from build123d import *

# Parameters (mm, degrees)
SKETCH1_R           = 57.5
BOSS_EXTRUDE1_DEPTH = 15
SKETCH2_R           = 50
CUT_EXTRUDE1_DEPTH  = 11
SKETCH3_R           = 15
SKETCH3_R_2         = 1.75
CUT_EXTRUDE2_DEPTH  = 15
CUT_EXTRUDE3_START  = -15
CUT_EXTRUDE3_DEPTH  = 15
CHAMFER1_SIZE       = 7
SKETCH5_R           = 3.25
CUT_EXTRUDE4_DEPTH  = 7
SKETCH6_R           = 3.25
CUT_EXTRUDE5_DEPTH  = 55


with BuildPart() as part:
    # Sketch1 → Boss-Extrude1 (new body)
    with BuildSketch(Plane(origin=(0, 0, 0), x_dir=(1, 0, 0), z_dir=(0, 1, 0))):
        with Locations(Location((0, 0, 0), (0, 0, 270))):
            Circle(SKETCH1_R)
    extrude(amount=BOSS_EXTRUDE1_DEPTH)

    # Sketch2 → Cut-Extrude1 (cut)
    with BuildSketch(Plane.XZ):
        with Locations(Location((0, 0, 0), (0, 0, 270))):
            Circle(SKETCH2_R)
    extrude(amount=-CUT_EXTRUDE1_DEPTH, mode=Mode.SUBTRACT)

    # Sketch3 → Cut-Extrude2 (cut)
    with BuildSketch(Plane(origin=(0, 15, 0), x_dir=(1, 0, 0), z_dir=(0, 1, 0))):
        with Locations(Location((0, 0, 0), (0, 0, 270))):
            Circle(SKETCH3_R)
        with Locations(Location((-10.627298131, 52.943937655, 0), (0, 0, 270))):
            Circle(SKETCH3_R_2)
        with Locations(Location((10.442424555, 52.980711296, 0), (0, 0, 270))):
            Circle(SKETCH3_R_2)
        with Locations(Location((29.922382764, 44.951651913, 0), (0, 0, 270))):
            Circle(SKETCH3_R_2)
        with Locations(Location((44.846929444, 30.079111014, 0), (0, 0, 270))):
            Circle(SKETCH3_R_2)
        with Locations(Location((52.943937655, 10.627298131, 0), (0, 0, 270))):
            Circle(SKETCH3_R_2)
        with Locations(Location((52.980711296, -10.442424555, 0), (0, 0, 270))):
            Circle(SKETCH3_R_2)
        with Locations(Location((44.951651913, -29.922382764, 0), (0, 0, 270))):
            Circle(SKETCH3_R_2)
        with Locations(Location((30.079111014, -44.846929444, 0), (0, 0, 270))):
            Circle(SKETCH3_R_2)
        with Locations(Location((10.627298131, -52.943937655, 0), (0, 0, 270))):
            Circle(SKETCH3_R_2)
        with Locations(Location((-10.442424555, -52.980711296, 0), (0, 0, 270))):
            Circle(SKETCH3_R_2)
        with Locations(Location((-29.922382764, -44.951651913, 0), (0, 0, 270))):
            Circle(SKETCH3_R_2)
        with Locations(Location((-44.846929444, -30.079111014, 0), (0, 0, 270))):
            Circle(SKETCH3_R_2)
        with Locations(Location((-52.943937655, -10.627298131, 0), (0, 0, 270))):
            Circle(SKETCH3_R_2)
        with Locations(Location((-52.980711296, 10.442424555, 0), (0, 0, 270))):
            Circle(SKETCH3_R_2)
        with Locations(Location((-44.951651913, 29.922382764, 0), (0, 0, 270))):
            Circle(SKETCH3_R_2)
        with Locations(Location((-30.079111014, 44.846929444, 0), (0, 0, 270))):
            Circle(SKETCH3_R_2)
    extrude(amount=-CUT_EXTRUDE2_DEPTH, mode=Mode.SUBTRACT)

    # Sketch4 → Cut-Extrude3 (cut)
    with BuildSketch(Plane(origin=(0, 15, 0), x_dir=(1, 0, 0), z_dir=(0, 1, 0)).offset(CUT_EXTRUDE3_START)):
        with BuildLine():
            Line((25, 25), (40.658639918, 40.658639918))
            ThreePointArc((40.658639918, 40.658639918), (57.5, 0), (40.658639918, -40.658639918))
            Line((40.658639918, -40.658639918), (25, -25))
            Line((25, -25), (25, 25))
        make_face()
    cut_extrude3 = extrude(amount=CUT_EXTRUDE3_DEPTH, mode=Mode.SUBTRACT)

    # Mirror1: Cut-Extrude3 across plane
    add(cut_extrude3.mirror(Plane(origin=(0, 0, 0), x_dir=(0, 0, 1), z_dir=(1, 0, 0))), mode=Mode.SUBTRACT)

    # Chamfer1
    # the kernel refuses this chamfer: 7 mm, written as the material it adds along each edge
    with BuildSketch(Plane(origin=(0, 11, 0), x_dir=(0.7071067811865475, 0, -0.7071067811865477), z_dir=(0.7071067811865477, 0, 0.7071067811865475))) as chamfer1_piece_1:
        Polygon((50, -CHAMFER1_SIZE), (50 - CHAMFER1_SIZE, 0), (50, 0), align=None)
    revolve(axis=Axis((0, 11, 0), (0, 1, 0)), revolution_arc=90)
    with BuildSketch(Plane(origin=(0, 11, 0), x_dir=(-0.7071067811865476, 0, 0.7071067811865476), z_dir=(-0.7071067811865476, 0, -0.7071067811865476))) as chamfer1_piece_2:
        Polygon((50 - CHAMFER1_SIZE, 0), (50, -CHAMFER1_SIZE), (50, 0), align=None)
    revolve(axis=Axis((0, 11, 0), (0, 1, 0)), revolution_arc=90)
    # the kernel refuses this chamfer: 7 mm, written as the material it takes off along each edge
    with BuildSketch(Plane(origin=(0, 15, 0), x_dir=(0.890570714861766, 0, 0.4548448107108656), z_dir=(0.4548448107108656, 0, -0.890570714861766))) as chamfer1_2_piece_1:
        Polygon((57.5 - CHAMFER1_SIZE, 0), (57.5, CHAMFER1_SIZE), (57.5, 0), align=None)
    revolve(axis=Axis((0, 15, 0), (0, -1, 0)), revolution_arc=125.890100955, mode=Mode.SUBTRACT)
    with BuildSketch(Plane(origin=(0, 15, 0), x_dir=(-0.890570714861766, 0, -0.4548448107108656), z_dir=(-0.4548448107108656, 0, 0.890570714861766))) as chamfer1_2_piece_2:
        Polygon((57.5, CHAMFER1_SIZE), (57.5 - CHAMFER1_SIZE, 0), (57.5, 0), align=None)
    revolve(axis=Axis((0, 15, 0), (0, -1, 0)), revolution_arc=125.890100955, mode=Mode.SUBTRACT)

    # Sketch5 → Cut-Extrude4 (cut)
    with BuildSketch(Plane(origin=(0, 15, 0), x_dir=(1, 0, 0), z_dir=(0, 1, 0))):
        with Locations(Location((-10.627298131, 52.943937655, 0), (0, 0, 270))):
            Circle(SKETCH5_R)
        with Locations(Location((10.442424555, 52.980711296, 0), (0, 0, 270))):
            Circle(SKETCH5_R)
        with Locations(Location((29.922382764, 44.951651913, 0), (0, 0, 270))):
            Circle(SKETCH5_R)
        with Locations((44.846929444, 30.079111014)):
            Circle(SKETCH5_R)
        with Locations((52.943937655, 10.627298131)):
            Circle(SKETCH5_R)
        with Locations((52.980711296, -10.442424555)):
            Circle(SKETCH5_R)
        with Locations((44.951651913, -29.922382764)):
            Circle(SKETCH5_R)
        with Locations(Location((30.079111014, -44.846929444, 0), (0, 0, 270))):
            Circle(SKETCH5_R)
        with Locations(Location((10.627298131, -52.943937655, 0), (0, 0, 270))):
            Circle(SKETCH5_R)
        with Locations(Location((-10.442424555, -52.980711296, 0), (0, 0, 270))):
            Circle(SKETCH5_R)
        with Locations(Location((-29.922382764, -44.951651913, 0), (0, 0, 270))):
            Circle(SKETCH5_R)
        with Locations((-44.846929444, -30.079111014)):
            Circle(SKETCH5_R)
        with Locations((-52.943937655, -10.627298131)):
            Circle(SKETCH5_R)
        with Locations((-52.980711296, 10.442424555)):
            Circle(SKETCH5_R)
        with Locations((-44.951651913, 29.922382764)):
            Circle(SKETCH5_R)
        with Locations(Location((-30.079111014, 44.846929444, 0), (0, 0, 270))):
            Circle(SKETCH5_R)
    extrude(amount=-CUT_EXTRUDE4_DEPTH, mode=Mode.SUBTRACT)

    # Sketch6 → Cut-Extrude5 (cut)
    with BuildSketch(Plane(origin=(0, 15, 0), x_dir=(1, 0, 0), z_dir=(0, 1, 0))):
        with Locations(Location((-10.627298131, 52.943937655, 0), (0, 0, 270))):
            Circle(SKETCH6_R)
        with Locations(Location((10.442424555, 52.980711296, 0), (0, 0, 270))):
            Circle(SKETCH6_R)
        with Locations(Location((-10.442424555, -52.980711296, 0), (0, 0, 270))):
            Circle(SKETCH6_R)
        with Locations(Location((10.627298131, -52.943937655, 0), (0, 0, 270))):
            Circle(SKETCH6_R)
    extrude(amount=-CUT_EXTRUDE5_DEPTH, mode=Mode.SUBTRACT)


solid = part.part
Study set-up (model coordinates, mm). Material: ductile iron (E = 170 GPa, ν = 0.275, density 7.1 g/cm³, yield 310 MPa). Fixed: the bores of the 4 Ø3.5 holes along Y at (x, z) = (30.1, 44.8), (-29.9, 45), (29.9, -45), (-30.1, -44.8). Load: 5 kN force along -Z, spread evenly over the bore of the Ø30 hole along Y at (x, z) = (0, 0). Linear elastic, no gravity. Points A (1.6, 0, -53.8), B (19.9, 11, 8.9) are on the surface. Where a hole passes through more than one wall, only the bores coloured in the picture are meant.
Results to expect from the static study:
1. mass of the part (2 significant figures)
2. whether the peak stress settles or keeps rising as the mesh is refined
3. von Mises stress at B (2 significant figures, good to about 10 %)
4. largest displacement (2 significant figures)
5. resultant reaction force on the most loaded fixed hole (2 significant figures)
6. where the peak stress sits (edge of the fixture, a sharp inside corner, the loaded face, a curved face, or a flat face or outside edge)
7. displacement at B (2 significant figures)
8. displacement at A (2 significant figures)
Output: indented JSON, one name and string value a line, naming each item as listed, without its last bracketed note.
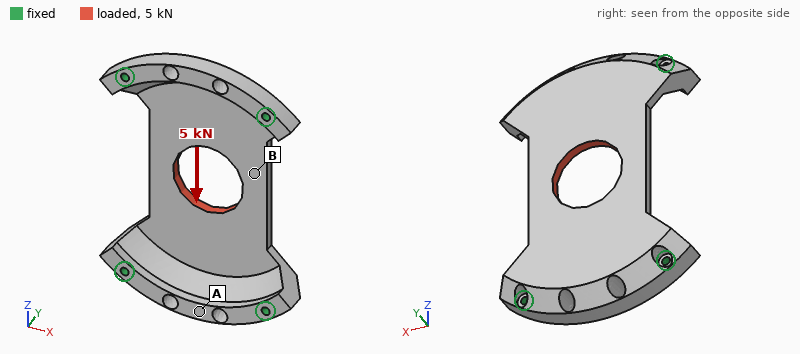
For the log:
{
  "mass of the part": "240 g",
  "whether the peak stress settles or keeps rising as the mesh is refined": "keeps rising",
  "von Mises stress at B": "19 MPa",
  "largest displacement": "14 µm",
  "resultant reaction force on the most loaded fixed hole": "1.3 kN",
  "where the peak stress sits": "edge of the fixture",
  "displacement at B": "12 µm",
  "displacement at A": "3.1 µm"
}
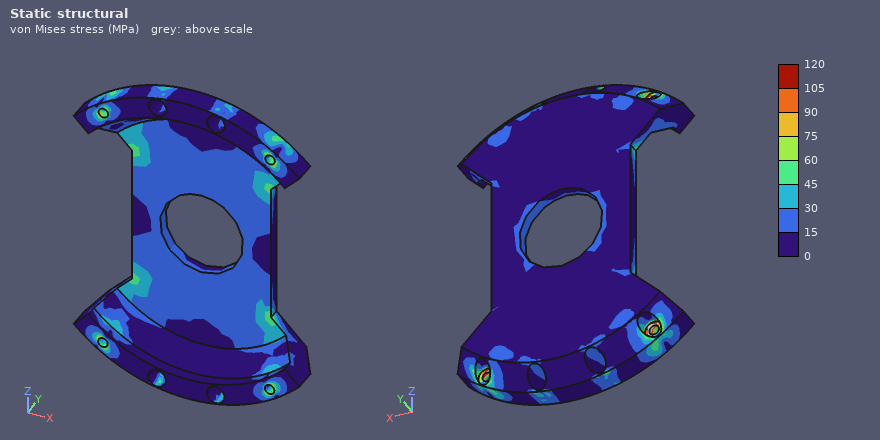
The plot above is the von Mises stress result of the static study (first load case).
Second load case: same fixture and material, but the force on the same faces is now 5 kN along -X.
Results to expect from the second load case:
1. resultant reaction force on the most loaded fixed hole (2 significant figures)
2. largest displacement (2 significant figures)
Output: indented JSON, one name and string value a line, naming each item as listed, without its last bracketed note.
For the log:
{
  "resultant reaction force on the most loaded fixed hole": "1.5 kN",
  "largest displacement": "18 µm"
}
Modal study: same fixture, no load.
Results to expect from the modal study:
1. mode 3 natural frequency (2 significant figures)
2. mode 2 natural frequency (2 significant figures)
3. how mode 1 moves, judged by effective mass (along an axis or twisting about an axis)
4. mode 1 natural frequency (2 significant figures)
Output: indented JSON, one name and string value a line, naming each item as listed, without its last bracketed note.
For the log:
{
  "mode 3 natural frequency": "5800 Hz",
  "mode 2 natural frequency": "4800 Hz",
  "how mode 1 moves, judged by effective mass": "along Y",
  "mode 1 natural frequency": "3300 Hz"
}
